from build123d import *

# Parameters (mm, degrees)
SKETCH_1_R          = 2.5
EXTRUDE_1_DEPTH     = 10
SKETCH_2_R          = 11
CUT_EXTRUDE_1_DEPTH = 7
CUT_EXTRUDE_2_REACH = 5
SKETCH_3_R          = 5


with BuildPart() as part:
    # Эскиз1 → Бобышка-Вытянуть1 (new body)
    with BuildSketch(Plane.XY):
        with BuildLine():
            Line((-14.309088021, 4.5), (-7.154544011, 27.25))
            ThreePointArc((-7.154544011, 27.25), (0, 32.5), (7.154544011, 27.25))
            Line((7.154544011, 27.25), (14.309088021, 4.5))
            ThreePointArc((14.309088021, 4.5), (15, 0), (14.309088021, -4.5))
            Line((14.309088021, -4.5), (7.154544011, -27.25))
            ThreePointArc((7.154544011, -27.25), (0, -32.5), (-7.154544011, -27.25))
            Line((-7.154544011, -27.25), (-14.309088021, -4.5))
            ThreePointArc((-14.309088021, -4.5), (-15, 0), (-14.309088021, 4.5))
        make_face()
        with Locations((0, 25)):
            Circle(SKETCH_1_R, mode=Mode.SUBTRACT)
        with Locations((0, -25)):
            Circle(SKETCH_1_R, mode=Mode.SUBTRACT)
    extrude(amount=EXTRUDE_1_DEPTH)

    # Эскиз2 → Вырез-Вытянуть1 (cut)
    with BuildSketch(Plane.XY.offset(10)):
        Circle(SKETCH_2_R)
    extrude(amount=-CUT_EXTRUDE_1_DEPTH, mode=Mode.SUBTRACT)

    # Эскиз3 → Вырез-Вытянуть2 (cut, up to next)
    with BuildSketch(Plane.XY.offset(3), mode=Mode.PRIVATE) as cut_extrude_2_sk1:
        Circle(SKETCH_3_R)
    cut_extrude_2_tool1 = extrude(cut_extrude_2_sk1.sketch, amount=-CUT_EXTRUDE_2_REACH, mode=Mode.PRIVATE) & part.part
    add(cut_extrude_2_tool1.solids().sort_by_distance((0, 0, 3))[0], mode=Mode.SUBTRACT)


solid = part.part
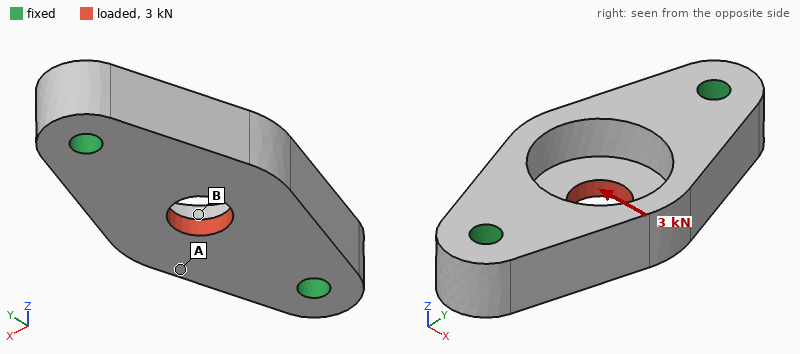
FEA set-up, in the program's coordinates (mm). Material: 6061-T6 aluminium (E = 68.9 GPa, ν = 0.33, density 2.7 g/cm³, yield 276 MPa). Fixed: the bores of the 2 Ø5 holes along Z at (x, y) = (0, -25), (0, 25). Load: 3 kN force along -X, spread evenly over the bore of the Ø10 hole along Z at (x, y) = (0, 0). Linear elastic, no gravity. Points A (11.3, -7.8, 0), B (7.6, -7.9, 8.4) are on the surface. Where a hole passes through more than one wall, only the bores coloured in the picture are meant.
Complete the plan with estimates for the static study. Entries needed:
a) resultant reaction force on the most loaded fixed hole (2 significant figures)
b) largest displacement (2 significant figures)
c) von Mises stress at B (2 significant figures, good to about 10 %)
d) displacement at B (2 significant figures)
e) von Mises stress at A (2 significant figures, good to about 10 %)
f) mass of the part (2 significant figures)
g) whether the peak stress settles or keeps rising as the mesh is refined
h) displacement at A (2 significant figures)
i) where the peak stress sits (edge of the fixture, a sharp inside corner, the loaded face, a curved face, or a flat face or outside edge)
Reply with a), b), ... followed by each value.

a) 1.5 kN
b) 22 µm
c) 10 MPa
d) 7.7 µm
e) 29 MPa
f) 28 g
g) keeps rising
h) 17 µm
i) edge of the fixture
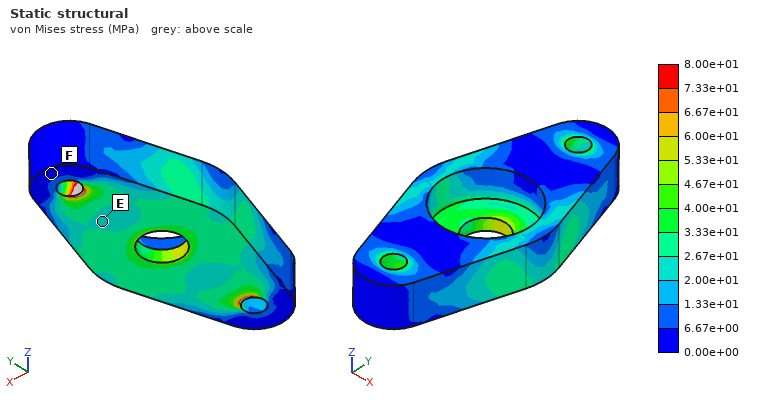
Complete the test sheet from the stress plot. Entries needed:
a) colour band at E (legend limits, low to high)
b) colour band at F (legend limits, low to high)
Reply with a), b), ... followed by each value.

a) 2.00e+01 to 2.67e+01 MPa
b) 0.00e+00 to 6.67e+00 MPa
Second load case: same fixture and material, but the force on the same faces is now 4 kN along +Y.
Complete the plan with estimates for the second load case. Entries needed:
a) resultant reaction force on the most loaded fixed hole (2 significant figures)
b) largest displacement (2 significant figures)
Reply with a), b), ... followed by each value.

a) 2.0 kN
b) 9.8 µm
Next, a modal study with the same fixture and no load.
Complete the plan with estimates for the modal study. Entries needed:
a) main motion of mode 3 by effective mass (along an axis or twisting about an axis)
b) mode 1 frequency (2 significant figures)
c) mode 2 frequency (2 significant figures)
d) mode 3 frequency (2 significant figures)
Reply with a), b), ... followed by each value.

a) along X
b) 16 kHz
c) 17 kHz
d) 24 kHz
